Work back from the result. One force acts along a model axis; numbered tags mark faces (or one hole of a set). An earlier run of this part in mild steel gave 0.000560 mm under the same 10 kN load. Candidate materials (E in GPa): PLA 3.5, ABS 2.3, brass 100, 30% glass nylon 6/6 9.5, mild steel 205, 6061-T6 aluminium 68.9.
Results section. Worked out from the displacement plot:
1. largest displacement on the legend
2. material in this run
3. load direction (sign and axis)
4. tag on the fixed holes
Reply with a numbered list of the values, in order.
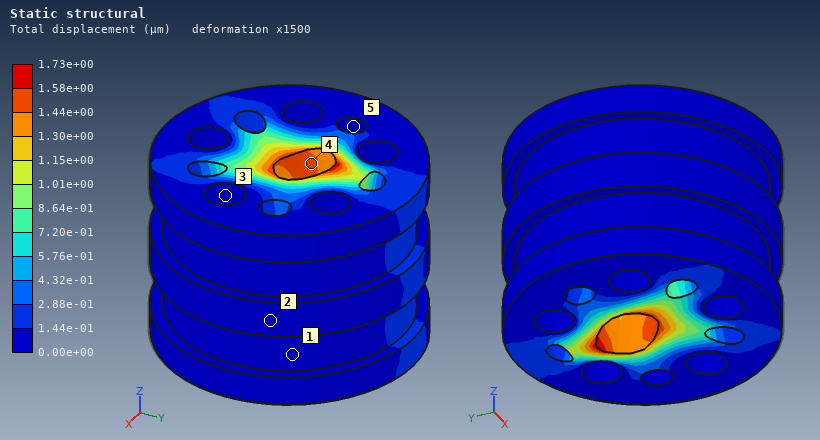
1. 1.73e+00 µm
2. 6061-T6 aluminium
3. +Y
4. 3
